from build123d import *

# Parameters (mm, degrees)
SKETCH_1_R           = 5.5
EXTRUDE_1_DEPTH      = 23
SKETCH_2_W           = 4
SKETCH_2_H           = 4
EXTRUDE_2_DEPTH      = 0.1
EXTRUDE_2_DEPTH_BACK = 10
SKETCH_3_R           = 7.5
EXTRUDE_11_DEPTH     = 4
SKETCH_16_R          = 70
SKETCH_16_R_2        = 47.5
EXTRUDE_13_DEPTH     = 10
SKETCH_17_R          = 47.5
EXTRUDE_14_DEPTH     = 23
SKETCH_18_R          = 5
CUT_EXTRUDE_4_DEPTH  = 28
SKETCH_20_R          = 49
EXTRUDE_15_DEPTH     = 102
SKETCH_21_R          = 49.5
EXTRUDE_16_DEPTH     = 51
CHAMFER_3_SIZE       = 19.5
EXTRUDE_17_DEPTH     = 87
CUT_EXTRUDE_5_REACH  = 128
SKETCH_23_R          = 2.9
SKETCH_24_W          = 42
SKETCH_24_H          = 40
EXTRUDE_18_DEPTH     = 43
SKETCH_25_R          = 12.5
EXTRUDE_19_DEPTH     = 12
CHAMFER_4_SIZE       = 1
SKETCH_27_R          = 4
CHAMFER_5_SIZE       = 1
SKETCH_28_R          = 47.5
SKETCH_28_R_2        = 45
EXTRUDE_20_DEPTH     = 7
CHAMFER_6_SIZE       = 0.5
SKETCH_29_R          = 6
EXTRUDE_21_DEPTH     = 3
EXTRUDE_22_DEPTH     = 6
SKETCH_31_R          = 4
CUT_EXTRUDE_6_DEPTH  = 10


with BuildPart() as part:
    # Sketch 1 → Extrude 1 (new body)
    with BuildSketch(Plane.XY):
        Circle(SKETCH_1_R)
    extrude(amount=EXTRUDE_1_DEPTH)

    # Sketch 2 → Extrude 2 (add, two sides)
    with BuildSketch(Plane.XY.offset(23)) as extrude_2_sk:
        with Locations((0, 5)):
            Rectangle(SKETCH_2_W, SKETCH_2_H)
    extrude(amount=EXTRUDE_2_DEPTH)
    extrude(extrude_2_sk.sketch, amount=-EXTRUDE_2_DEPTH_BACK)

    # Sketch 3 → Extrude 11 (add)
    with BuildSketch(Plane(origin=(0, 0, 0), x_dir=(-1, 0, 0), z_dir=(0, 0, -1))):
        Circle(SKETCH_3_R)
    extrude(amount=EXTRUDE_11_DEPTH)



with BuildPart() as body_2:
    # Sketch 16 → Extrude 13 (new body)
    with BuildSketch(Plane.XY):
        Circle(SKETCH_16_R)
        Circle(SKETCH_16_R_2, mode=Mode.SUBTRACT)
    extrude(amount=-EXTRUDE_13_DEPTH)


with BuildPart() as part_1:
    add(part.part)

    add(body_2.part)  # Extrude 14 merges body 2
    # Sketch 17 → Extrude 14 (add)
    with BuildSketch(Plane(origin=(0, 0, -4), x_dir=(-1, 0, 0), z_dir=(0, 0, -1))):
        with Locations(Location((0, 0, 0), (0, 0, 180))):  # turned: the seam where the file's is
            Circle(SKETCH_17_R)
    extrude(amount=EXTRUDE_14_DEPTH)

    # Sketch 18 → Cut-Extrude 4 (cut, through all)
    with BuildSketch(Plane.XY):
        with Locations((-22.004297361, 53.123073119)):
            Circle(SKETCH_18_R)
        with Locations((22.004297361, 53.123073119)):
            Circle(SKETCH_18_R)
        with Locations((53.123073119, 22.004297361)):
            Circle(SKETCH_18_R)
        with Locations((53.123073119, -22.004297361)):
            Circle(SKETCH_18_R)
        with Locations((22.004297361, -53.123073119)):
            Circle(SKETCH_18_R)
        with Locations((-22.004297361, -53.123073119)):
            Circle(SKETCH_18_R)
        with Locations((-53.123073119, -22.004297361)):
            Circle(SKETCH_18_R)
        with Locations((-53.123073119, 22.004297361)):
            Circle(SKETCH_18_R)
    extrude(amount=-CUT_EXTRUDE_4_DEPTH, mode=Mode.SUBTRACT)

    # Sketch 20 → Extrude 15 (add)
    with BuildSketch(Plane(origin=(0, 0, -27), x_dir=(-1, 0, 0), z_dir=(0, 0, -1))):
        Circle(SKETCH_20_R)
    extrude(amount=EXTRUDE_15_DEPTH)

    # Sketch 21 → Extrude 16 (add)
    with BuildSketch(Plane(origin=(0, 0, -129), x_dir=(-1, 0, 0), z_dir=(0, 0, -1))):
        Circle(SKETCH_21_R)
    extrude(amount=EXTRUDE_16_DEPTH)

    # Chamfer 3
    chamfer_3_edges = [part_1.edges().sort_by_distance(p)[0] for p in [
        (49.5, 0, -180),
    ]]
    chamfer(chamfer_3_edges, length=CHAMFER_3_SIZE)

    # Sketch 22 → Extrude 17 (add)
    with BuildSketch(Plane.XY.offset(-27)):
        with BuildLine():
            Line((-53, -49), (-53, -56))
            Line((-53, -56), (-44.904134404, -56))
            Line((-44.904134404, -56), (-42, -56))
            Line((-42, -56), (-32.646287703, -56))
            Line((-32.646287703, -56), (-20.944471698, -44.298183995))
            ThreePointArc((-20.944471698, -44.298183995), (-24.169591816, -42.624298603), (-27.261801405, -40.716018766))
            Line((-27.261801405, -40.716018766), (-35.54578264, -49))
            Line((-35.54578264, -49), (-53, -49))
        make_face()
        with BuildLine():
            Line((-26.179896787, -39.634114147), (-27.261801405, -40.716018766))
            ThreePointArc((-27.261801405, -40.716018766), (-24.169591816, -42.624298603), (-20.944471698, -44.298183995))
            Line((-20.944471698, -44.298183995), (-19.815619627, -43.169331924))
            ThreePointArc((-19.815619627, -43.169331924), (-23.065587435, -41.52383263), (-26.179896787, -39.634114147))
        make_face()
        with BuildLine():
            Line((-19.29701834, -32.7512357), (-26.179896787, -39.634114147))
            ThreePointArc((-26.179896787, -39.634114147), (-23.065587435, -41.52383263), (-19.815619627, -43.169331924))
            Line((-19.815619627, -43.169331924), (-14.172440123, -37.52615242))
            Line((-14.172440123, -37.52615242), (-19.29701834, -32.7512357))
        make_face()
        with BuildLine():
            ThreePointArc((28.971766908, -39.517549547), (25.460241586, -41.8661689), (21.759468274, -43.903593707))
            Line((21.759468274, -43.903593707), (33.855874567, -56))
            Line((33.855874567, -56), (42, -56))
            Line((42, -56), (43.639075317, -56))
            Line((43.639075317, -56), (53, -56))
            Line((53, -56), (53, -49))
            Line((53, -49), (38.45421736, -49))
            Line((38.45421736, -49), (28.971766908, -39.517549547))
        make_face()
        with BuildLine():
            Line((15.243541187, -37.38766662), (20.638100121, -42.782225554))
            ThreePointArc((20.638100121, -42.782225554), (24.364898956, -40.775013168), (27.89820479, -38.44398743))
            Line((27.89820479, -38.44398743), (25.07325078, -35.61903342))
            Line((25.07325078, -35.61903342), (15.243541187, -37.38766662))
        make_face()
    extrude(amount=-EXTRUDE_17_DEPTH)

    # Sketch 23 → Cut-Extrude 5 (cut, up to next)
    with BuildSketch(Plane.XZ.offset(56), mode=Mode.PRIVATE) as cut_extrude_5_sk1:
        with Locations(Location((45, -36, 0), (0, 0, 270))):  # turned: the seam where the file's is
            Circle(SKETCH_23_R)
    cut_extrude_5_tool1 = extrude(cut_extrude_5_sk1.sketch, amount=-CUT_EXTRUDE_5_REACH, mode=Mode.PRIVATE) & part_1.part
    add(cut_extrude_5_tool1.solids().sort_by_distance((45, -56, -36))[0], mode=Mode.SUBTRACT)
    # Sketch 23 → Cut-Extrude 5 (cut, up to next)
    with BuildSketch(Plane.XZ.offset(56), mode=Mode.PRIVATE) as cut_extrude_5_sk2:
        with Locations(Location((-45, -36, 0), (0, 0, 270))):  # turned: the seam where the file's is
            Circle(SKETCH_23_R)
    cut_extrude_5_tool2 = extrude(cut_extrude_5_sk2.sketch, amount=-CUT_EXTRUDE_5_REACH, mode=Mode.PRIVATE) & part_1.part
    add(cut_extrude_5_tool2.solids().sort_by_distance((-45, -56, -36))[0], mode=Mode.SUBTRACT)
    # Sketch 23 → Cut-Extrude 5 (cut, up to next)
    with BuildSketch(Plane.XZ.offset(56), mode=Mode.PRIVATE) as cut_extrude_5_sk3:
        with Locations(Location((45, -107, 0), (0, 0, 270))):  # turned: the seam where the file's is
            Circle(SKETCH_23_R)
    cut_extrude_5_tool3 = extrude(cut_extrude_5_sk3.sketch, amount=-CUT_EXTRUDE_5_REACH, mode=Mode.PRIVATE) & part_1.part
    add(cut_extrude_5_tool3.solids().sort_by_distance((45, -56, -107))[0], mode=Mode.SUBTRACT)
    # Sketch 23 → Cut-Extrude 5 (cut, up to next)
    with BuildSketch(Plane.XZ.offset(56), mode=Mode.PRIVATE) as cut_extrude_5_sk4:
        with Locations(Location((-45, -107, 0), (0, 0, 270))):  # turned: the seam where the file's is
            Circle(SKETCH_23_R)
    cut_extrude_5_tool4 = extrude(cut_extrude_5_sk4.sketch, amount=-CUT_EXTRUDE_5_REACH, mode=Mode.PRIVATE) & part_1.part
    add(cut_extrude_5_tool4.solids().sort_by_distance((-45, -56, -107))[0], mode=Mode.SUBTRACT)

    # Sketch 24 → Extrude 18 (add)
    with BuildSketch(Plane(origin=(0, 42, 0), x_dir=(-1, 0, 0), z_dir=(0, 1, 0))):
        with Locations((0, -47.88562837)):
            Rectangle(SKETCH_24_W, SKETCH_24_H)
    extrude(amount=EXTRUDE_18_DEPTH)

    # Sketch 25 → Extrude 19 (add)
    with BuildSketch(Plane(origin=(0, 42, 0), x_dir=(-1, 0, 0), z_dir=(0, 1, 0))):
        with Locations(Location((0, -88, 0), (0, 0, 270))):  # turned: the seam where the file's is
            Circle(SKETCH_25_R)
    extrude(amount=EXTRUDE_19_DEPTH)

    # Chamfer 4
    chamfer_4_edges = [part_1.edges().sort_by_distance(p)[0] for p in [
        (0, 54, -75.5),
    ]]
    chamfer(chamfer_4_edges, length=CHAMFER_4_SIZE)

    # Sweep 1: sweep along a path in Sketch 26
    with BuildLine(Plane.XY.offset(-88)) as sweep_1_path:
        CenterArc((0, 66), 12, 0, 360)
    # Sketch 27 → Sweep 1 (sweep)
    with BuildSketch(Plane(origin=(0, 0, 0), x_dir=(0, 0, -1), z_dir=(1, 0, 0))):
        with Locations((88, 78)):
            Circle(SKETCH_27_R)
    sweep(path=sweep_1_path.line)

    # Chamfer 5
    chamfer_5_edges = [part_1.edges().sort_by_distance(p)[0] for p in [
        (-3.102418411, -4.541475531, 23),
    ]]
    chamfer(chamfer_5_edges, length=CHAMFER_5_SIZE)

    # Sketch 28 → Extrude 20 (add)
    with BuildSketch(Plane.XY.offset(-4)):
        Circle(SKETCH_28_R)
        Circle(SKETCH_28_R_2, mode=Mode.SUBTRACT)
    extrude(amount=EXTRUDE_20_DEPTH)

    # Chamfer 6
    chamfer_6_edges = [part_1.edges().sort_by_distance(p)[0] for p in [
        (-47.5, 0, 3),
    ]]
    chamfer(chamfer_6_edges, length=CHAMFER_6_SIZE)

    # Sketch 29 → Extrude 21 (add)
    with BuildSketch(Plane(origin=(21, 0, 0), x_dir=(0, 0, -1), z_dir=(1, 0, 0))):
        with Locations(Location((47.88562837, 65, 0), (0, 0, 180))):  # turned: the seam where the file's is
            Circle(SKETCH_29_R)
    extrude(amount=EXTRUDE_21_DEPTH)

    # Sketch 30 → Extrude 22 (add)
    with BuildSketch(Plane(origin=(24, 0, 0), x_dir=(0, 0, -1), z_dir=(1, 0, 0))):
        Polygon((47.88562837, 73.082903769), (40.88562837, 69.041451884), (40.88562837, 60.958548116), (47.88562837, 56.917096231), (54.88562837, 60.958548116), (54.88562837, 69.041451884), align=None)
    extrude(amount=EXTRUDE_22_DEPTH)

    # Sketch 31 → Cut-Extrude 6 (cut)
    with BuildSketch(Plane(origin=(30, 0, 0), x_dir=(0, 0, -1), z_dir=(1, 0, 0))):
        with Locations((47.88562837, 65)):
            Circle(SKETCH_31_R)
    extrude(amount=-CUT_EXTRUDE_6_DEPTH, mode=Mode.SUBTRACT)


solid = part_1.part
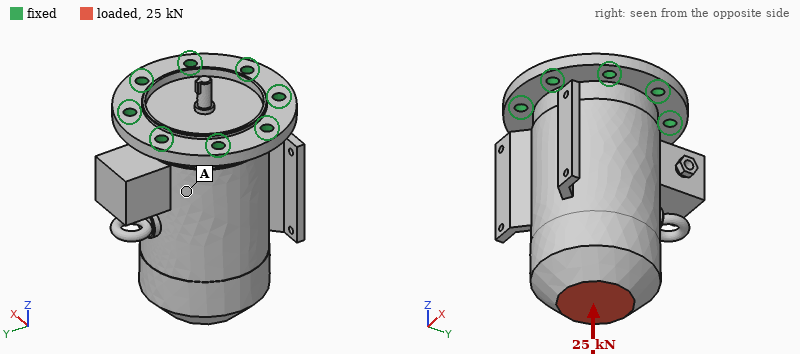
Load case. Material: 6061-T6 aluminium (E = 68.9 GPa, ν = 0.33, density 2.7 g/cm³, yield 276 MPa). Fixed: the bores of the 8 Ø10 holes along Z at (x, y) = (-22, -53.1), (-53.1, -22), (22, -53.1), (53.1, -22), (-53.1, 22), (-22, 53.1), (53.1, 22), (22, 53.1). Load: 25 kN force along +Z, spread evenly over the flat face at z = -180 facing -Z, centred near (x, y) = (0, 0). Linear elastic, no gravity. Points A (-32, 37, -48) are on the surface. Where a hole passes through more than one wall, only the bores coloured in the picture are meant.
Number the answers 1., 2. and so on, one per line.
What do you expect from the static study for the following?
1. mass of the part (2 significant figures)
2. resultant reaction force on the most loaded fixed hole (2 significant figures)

1. 4.0 kg
2. 3.6 kN
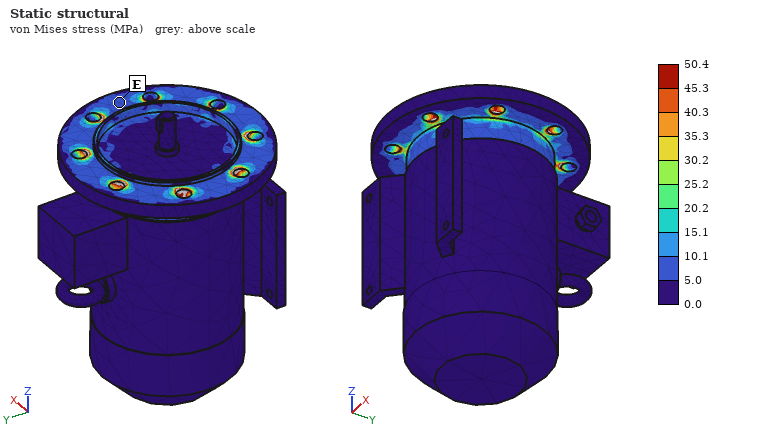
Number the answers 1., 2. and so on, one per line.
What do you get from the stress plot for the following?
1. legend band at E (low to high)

1. 5.0 to 10.1 MPa
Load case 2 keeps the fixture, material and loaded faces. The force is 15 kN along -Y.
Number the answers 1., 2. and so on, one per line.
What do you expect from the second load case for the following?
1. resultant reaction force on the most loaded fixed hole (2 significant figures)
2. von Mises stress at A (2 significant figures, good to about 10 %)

1. 13 kN
2. 15 MPa
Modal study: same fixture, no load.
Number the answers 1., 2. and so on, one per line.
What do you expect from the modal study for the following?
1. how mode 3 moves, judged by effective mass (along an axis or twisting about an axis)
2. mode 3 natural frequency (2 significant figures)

1. along Z
2. 3700 Hz
